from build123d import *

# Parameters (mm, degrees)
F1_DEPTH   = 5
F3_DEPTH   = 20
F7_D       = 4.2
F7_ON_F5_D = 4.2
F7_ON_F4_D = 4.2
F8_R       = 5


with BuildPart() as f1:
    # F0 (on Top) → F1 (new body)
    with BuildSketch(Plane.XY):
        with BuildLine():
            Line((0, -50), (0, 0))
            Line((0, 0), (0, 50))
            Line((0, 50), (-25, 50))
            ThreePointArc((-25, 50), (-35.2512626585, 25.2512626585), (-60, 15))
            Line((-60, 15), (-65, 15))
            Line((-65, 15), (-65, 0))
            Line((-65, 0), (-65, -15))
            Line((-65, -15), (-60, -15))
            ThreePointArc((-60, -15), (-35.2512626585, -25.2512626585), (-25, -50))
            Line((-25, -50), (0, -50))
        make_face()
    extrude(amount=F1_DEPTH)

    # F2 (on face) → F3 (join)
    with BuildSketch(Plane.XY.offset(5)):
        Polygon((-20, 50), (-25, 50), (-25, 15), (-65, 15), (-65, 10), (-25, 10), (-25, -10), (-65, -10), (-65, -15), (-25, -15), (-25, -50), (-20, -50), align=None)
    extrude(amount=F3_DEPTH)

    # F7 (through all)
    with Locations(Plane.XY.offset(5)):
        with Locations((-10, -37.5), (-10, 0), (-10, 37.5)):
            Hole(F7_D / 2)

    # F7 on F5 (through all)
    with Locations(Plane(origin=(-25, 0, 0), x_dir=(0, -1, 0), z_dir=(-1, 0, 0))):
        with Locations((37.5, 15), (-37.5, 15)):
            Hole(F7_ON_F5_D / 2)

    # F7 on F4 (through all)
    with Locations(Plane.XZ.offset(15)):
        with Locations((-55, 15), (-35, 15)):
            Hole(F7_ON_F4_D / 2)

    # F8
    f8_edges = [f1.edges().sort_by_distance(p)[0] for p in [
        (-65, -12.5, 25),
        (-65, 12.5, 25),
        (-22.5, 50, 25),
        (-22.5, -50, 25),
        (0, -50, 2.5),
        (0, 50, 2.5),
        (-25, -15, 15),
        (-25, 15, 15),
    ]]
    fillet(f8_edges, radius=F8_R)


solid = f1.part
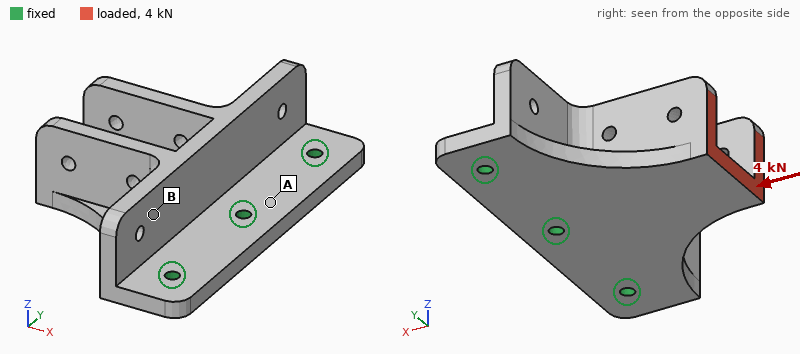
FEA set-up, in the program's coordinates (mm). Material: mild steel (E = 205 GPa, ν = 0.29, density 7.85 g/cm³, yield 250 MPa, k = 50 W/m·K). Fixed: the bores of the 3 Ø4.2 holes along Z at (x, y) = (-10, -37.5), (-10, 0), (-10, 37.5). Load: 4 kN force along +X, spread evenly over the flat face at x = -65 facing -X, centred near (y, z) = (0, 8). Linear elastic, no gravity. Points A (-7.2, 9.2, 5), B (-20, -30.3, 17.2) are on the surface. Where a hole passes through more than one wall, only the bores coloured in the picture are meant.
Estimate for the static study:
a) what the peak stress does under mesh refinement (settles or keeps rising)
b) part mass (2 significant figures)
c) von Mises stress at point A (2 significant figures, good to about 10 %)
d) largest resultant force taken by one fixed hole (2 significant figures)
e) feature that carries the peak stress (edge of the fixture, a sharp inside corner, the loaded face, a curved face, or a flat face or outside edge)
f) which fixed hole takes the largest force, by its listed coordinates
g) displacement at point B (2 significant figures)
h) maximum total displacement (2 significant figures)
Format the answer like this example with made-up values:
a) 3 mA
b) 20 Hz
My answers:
a) keeps rising
b) 300 g
c) 23 MPa
d) 2.5 kN
e) edge of the fixture
f) (-10, 0)
g) 22 µm
h) 85 µm
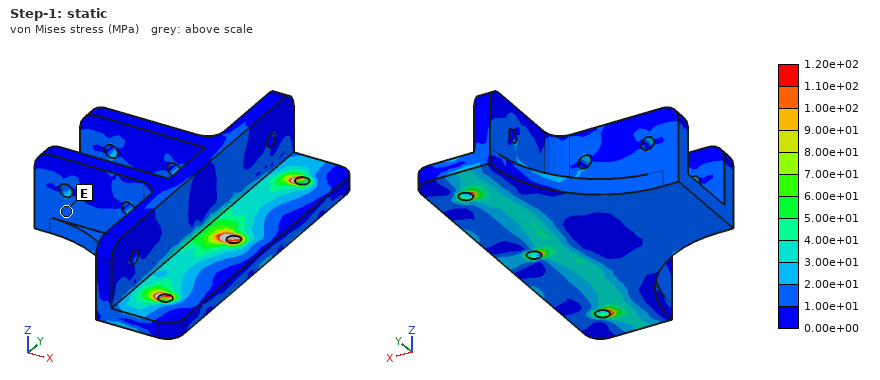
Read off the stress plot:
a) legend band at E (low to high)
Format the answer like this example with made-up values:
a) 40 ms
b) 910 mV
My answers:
a) 1.00e+01 to 2.00e+01 MPa
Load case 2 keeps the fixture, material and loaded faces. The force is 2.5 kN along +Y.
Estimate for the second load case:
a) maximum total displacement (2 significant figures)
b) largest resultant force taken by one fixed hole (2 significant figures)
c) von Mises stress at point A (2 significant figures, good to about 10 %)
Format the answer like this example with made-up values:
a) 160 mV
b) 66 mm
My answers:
a) 50 µm
b) 2.1 kN
c) 6.4 MPa
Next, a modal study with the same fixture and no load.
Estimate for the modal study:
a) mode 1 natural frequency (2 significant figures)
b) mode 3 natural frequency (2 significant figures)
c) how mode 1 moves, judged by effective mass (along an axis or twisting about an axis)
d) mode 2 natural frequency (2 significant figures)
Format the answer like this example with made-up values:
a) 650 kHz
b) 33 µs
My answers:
a) 1500 Hz
b) 7500 Hz
c) along Z
d) 4600 Hz
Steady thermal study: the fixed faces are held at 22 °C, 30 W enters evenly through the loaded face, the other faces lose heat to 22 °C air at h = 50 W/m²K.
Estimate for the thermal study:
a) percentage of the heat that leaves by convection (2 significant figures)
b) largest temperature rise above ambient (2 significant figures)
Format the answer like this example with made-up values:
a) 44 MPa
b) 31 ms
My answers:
a) 53 %
b) 68 K
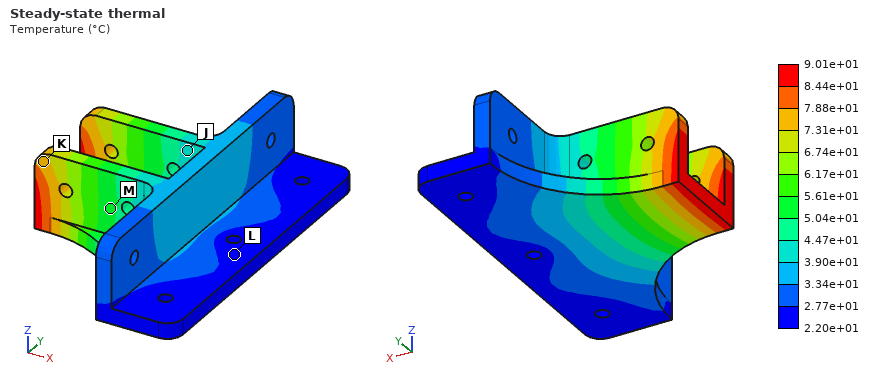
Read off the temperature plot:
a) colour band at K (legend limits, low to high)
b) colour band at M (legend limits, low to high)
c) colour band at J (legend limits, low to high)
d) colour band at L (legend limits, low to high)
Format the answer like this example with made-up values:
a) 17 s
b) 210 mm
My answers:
a) 7.31e+01 to 7.88e+01 °C
b) 5.04e+01 to 5.61e+01 °C
c) 3.90e+01 to 4.47e+01 °C
d) 2.20e+01 to 2.77e+01 °C
